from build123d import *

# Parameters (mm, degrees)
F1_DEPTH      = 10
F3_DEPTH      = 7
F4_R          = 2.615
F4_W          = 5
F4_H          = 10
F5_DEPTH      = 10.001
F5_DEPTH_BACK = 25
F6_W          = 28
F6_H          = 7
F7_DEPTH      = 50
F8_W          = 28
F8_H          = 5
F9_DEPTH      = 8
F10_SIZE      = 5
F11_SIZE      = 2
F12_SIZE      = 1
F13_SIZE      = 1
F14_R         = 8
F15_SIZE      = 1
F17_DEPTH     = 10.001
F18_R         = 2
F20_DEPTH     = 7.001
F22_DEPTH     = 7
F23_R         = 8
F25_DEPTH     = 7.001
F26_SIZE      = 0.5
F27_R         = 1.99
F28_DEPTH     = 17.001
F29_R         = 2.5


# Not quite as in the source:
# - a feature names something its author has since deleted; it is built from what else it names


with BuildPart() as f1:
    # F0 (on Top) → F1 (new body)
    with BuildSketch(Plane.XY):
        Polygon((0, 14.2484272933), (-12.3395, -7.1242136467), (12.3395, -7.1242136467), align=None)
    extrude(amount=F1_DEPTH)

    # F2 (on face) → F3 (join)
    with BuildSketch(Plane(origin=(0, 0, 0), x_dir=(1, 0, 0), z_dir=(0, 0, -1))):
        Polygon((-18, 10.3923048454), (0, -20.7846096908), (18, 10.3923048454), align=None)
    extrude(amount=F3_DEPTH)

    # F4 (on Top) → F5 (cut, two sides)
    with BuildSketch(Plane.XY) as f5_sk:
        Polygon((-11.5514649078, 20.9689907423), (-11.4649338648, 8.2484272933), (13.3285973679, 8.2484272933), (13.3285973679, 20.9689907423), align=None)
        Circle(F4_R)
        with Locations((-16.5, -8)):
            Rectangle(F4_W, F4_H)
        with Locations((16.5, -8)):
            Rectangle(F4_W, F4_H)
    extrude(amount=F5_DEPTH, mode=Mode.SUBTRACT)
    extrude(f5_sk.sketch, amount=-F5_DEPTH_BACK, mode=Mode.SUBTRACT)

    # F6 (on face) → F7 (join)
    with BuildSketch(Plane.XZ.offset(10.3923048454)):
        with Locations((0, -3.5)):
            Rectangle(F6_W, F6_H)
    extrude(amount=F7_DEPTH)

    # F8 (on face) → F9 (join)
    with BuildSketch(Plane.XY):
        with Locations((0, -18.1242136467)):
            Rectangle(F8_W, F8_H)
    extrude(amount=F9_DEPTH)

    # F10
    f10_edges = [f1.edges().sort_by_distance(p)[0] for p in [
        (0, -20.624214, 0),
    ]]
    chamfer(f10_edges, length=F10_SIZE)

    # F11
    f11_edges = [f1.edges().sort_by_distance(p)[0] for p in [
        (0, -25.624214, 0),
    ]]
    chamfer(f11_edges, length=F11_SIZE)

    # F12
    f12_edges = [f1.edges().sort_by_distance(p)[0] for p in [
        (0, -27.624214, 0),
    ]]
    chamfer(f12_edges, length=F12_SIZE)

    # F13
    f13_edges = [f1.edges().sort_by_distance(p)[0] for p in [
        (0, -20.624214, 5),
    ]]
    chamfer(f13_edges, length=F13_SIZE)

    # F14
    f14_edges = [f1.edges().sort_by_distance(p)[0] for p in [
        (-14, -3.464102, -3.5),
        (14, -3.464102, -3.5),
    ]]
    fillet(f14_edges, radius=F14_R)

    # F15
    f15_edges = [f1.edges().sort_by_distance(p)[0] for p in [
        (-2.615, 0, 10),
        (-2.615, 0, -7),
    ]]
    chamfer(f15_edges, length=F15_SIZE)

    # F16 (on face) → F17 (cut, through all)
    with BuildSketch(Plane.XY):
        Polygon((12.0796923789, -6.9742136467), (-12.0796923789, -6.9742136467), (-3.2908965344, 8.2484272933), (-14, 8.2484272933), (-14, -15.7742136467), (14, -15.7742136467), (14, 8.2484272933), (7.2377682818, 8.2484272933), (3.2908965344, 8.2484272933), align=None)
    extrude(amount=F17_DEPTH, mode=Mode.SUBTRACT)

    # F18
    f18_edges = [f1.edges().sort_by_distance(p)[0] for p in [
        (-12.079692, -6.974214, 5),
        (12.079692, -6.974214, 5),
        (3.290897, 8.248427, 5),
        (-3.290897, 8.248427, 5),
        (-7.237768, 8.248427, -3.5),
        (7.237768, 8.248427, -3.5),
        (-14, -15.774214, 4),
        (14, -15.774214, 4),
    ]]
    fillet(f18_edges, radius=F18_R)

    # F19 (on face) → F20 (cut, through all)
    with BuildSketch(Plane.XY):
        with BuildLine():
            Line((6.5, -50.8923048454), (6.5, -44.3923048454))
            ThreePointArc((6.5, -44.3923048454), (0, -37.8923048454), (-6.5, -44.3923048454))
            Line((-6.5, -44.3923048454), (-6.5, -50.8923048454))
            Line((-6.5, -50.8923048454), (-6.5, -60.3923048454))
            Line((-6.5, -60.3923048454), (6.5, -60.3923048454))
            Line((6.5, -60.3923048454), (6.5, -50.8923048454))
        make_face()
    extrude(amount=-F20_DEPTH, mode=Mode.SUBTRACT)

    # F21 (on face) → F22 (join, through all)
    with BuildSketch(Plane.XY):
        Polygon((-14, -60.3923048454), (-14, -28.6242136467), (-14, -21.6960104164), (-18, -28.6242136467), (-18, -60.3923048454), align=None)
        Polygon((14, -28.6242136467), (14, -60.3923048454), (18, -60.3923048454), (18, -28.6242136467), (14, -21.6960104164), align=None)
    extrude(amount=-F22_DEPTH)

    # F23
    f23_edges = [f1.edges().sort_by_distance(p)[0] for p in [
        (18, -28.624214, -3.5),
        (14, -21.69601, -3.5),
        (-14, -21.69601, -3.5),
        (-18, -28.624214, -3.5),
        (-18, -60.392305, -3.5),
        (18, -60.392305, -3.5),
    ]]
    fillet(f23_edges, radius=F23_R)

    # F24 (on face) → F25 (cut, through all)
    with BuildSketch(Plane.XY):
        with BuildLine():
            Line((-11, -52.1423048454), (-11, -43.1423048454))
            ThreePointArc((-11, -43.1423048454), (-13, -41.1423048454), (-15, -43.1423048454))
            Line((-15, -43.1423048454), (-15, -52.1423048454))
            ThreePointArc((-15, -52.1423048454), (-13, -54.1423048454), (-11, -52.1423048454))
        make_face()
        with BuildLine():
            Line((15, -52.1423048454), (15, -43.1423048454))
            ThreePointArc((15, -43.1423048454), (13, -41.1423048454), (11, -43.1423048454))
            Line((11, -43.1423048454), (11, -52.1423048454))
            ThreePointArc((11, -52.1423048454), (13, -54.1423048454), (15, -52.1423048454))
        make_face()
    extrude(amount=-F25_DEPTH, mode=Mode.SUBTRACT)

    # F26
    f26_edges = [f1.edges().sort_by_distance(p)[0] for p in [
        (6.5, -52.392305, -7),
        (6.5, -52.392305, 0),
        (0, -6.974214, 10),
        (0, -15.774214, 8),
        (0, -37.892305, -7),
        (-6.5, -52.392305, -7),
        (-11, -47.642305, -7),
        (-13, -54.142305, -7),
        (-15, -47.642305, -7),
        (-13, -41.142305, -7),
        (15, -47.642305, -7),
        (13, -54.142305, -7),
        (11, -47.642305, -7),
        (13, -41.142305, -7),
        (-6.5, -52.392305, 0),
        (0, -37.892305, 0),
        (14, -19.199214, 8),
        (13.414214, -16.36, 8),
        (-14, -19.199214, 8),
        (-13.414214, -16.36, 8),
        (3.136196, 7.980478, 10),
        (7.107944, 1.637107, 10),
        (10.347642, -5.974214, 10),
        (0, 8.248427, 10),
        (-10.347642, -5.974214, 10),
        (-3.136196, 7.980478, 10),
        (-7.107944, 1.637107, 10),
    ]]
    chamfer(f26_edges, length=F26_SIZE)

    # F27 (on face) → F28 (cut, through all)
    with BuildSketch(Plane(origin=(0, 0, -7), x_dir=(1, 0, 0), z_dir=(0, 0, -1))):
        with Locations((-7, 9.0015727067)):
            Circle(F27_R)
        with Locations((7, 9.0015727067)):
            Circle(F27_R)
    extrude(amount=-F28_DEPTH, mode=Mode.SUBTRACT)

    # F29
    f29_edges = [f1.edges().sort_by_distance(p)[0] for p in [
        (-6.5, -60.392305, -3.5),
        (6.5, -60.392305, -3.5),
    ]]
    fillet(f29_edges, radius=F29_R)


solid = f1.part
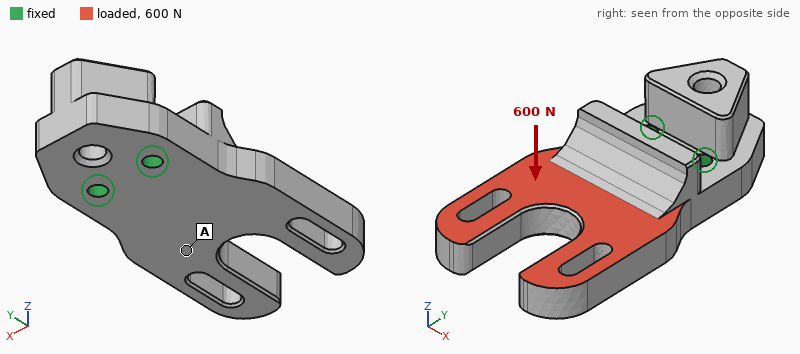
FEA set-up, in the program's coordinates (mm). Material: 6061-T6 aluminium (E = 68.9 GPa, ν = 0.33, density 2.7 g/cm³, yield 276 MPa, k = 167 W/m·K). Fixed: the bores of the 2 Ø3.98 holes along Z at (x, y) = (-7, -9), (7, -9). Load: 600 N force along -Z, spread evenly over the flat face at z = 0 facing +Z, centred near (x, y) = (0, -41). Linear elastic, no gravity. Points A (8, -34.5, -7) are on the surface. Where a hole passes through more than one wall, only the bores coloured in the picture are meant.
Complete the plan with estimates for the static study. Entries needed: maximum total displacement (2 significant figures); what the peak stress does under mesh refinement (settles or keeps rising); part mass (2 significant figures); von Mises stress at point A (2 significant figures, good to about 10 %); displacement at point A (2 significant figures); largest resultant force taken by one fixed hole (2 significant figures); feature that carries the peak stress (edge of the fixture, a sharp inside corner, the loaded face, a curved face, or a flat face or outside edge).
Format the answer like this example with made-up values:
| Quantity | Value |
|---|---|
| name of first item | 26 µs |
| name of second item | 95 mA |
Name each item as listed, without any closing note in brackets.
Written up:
| Quantity | Value |
|---|---|
| maximum total displacement | 0.19 mm |
| what the peak stress does under mesh refinement | keeps rising |
| part mass | 41 g |
| von Mises stress at point A | 16 MPa |
| displacement at point A | 0.071 mm |
| largest resultant force taken by one fixed hole | 300 N |
| feature that carries the peak stress | edge of the fixture |
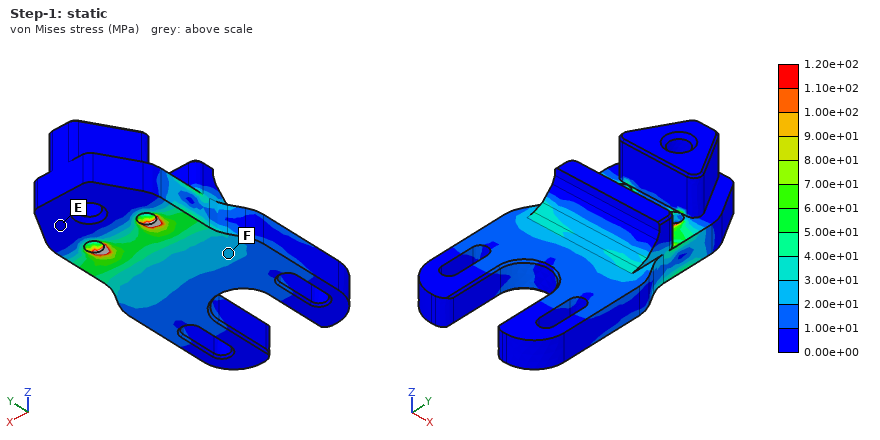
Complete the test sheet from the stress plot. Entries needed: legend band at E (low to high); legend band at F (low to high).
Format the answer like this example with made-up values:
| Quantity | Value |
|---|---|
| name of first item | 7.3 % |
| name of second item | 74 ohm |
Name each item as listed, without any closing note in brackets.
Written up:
| Quantity | Value |
|---|---|
| legend band at E | 0.00e+00 to 1.00e+01 MPa |
| legend band at F | 2.00e+01 to 3.00e+01 MPa |
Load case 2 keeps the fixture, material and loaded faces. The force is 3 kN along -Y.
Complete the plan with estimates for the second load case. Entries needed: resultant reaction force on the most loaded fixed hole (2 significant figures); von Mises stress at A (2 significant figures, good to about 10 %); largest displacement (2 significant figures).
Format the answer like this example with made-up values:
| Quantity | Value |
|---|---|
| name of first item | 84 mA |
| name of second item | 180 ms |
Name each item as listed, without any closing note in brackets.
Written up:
| Quantity | Value |
|---|---|
| resultant reaction force on the most loaded fixed hole | 1.5 kN |
| von Mises stress at A | 15 MPa |
| largest displacement | 0.17 mm |
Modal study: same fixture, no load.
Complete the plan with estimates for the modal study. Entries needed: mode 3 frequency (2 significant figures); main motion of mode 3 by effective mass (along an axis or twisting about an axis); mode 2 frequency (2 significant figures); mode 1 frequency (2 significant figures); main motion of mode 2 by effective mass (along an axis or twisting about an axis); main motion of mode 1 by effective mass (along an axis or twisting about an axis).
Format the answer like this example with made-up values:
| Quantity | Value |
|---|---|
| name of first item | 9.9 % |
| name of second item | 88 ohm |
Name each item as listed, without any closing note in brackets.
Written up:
| Quantity | Value |
|---|---|
| mode 3 frequency | 7000 Hz |
| main motion of mode 3 by effective mass | along X |
| mode 2 frequency | 5300 Hz |
| mode 1 frequency | 2900 Hz |
| main motion of mode 2 by effective mass | twisting about Y |
| main motion of mode 1 by effective mass | along Z |
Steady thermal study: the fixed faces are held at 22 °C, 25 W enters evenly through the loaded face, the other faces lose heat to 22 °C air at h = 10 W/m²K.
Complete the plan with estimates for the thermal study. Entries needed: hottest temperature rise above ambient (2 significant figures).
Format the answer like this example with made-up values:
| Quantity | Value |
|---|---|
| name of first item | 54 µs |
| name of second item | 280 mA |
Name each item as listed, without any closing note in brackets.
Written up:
| Quantity | Value |
|---|---|
| hottest temperature rise above ambient | 24 K |
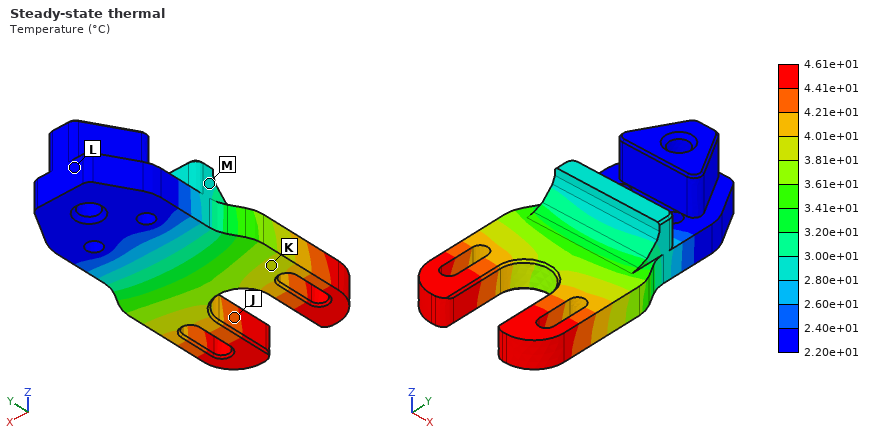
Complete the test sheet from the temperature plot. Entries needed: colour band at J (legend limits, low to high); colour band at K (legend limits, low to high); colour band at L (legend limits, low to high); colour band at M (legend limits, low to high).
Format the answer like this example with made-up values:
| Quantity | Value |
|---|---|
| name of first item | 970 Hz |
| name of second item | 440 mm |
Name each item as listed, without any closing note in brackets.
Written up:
| Quantity | Value |
|---|---|
| colour band at J | 4.21e+01 to 4.41e+01 °C |
| colour band at K | 3.81e+01 to 4.01e+01 °C |
| colour band at L | 2.20e+01 to 2.40e+01 °C |
| colour band at M | 2.80e+01 to 3.00e+01 °C |
